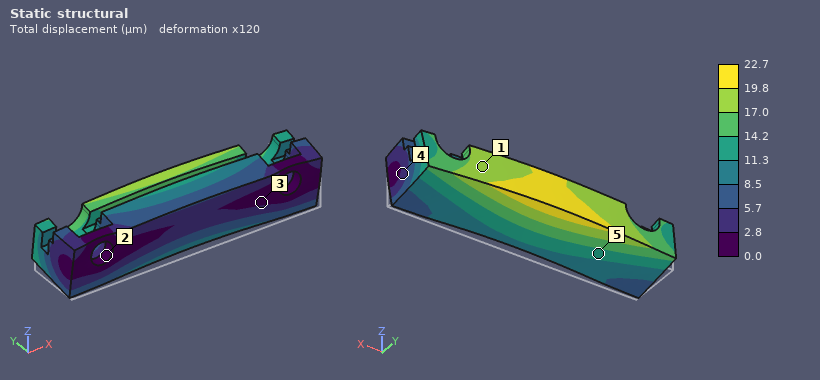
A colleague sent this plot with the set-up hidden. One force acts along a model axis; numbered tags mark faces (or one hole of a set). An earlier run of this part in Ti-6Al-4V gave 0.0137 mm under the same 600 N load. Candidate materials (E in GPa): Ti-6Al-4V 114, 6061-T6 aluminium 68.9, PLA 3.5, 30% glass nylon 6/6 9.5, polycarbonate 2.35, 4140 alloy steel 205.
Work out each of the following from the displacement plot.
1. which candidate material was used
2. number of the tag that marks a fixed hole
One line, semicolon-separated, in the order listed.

6061-T6 aluminium; 2
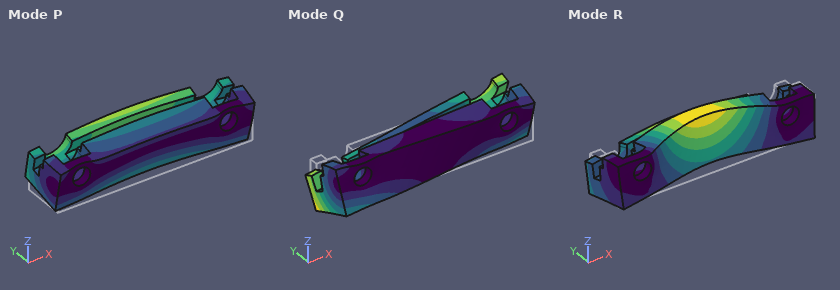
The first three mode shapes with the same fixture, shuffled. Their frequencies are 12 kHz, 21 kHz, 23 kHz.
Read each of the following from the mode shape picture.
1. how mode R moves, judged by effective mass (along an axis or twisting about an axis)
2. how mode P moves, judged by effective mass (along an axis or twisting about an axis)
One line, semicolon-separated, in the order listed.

along Y; along Z
